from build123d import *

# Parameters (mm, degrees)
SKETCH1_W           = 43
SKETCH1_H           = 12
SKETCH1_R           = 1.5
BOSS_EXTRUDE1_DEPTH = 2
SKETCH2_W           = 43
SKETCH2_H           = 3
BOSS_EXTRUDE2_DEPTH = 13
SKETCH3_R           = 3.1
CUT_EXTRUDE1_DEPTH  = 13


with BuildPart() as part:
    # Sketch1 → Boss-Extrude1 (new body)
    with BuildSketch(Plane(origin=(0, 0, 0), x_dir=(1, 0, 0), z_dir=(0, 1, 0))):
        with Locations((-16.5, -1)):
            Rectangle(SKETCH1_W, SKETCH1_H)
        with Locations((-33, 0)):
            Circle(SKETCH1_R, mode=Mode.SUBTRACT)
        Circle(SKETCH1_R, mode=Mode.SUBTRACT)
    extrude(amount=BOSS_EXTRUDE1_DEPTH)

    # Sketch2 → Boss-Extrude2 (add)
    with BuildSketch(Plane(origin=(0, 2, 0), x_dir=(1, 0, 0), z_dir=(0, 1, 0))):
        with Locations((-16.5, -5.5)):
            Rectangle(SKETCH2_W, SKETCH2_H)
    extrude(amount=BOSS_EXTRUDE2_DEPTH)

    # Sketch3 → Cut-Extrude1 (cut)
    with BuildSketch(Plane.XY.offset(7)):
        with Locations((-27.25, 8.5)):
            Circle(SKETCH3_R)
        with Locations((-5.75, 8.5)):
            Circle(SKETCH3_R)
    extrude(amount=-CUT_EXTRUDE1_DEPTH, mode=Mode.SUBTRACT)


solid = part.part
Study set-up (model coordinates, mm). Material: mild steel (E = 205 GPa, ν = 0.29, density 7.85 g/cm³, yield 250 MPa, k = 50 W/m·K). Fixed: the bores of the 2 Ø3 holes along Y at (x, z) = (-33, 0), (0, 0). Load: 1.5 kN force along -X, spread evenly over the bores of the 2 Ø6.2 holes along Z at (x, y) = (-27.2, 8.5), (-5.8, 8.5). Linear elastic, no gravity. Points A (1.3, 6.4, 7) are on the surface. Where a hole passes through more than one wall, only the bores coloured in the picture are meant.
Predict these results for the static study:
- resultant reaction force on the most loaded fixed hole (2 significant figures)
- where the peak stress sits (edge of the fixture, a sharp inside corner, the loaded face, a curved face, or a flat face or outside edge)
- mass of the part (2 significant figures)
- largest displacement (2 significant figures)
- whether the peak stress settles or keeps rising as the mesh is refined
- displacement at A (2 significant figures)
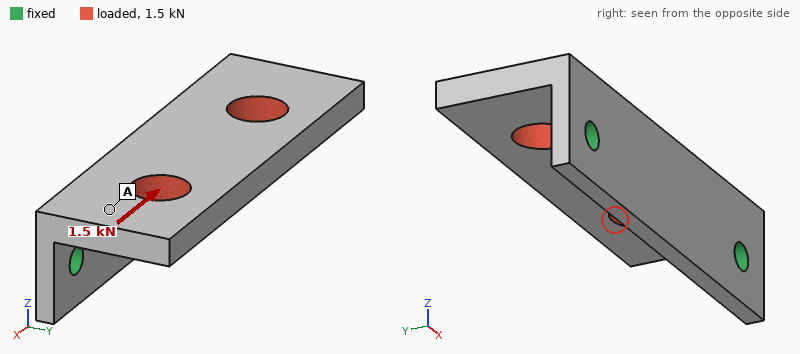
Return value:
850 N
edge of the fixture
20 g
18 µm
keeps rising
10.0 µm
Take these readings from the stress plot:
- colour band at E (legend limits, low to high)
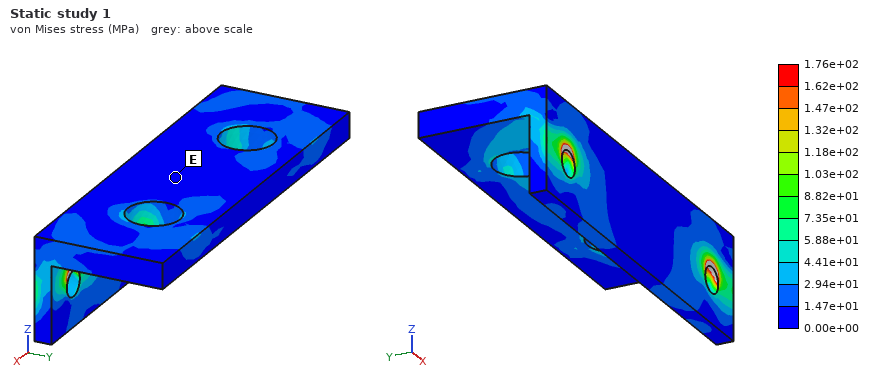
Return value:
0.00e+00 to 1.47e+01 MPa
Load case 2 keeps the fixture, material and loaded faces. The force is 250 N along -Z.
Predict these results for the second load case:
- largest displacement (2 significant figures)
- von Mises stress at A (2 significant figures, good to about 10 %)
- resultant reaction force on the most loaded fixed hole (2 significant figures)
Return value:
35 µm
18 MPa
130 N
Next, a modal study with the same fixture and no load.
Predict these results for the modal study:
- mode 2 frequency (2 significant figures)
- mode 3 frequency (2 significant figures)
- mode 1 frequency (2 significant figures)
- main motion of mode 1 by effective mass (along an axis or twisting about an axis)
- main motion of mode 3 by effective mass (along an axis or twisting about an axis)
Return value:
8900 Hz
14 kHz
4500 Hz
along Z
along Y
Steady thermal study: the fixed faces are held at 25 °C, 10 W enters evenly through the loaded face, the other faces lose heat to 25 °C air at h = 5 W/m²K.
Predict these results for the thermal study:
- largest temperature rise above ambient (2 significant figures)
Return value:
39 K
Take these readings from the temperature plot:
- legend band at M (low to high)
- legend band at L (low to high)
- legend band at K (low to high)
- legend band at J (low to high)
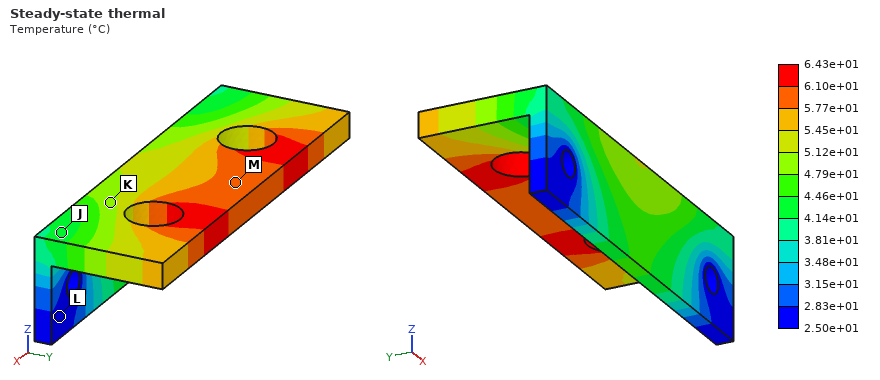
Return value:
5.77e+01 to 6.10e+01 °C
2.50e+01 to 2.83e+01 °C
4.79e+01 to 5.12e+01 °C
4.14e+01 to 4.46e+01 °C
